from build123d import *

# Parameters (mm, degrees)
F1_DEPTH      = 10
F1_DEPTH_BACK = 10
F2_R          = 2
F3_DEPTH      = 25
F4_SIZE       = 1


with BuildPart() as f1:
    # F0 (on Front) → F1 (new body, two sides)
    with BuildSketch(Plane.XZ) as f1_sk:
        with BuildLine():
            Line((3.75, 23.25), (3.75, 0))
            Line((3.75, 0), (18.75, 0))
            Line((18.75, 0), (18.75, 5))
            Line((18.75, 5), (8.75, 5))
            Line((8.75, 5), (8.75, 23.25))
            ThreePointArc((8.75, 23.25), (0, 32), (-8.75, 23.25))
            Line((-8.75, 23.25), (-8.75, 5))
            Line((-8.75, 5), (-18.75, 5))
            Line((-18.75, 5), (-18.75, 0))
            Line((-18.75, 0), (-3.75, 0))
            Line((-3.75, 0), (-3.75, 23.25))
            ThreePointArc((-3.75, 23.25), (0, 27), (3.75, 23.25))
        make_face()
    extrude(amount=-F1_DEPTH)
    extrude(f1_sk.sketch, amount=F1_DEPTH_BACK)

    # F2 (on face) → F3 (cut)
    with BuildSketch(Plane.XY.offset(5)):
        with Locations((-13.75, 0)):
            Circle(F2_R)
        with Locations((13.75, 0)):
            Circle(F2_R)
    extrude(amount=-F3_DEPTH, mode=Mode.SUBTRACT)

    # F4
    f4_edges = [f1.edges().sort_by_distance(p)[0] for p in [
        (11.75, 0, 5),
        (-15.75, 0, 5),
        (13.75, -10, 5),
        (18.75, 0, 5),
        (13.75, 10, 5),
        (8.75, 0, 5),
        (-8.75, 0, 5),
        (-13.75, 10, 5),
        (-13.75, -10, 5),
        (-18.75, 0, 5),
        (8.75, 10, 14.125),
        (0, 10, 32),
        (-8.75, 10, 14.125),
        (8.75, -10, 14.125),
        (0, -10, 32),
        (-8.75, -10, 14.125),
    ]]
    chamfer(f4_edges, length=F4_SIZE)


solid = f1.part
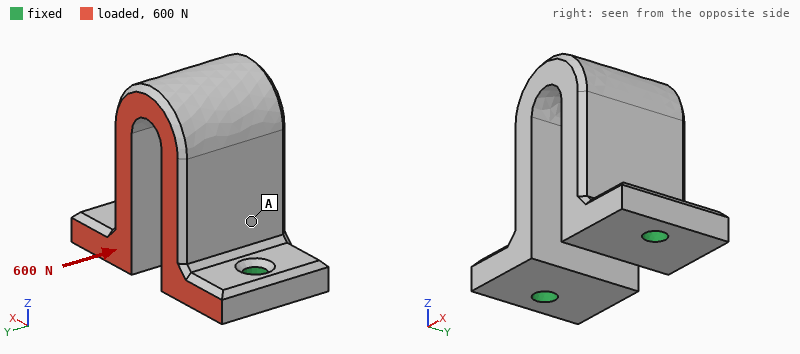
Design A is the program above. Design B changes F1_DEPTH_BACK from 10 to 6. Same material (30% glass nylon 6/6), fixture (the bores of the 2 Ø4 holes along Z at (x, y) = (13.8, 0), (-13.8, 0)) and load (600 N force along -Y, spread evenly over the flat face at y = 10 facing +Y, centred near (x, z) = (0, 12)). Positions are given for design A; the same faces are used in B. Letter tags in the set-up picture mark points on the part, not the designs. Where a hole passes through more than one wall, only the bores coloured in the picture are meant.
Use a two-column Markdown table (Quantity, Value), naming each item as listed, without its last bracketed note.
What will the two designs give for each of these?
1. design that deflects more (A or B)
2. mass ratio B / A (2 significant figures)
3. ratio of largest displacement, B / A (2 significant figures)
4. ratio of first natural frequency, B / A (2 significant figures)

| Quantity | Value |
|---|---|
| design that deflects more | B |
| mass ratio B / A | 0.79 |
| ratio of largest displacement, B / A | 1.2 |
| ratio of first natural frequency, B / A | 1.0 |
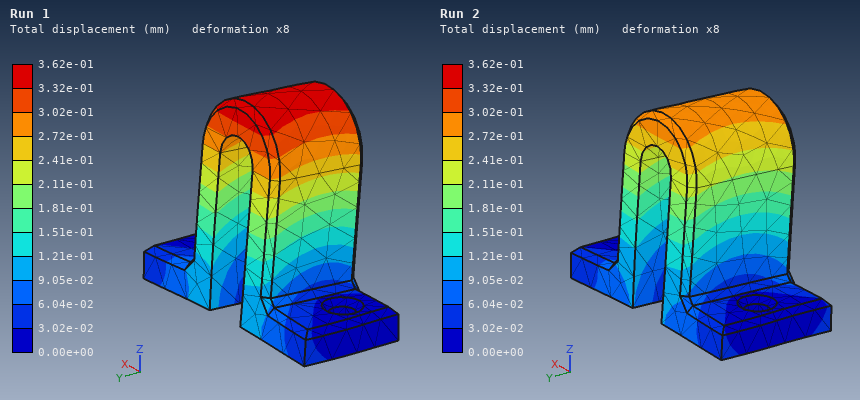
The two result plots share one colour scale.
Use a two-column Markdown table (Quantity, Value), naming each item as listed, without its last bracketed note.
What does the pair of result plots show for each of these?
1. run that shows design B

| Quantity | Value |
|---|---|
| run that shows design B | Run 1 |
